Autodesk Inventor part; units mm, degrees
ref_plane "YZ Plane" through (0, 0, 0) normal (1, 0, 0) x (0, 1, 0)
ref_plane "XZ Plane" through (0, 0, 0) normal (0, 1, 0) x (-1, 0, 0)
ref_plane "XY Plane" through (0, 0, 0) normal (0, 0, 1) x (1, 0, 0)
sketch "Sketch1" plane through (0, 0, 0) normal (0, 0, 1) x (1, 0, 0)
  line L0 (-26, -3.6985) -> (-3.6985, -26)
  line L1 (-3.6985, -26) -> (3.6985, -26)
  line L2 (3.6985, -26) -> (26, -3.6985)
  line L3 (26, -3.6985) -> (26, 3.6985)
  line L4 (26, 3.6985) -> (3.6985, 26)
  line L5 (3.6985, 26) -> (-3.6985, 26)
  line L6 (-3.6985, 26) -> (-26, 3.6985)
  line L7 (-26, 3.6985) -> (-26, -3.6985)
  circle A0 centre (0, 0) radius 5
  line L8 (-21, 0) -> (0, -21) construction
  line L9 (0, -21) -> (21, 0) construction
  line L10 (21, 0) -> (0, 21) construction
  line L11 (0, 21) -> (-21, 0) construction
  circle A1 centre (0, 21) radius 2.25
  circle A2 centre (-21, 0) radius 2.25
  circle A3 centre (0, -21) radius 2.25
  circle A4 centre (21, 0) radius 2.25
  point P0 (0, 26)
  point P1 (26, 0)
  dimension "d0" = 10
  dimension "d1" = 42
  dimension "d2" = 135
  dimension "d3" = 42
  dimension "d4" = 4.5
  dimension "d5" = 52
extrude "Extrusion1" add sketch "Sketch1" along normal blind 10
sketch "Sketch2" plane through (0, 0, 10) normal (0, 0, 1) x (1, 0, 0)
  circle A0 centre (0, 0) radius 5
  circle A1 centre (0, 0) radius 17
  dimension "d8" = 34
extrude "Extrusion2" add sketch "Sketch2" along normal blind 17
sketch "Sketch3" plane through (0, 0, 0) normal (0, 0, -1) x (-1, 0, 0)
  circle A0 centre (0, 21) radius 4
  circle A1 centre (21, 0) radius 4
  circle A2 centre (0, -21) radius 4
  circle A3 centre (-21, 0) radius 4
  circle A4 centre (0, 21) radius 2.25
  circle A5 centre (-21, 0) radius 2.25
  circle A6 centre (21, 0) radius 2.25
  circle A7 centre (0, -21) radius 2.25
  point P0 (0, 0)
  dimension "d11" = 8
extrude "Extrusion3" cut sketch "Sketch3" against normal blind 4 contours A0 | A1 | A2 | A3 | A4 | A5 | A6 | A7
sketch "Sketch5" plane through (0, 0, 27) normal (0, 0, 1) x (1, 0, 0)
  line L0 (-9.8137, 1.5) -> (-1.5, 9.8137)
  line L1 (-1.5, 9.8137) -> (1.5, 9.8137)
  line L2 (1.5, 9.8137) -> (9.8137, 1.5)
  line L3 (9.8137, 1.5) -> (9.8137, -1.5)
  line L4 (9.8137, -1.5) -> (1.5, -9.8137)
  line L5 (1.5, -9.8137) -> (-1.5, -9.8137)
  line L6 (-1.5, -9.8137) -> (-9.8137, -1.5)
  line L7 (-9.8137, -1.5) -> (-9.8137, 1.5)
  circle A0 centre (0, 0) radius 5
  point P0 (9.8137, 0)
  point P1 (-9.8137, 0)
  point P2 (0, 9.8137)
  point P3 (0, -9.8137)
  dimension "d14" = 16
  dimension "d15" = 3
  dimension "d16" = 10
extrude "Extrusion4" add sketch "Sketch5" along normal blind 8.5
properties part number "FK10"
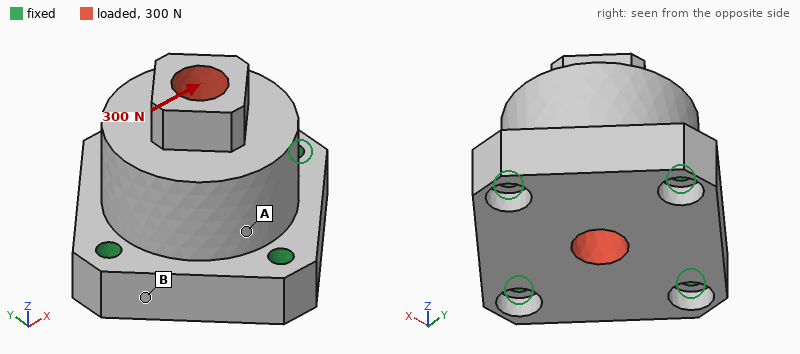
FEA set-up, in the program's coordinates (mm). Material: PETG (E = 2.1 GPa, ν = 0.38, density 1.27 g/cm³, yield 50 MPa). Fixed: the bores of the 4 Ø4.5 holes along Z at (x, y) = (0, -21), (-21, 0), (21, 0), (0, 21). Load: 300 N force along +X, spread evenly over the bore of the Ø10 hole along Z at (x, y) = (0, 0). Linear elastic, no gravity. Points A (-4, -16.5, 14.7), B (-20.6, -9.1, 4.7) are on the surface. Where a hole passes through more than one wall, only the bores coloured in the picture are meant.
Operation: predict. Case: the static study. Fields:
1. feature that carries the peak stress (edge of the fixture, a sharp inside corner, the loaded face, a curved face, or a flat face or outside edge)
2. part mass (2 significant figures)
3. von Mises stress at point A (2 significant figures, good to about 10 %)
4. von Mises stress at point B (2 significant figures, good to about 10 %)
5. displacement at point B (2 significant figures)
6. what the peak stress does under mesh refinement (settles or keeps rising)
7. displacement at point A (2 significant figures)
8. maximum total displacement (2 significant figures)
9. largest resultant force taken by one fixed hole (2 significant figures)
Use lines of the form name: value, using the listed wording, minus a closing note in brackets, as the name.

feature that carries the peak stress: edge of the fixture
part mass: 39 g
von Mises stress at point A: 0.35 MPa
von Mises stress at point B: 0.65 MPa
displacement at point B: 6.0 µm
what the peak stress does under mesh refinement: keeps rising
displacement at point A: 8.5 µm
maximum total displacement: 31 µm
largest resultant force taken by one fixed hole: 130 N
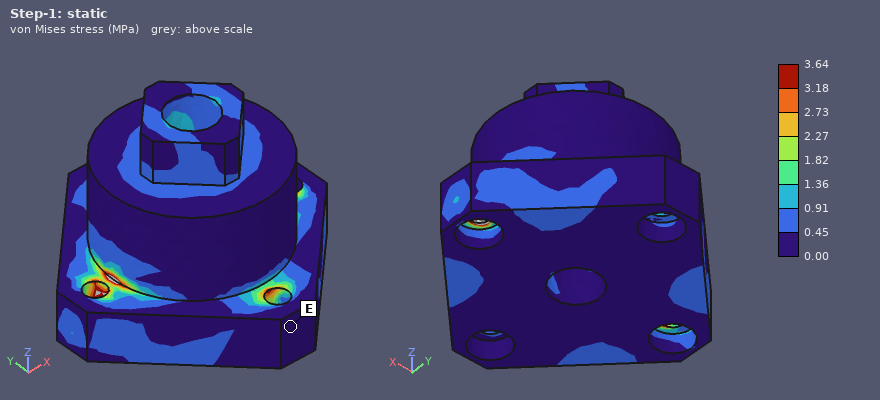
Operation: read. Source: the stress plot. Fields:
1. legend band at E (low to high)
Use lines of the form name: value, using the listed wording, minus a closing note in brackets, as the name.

legend band at E: 0.00 to 0.45 MPa
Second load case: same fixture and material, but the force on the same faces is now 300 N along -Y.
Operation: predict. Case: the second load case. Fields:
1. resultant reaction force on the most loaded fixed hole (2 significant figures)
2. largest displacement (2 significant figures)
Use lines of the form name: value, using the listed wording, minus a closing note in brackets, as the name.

resultant reaction force on the most loaded fixed hole: 130 N
largest displacement: 31 µm
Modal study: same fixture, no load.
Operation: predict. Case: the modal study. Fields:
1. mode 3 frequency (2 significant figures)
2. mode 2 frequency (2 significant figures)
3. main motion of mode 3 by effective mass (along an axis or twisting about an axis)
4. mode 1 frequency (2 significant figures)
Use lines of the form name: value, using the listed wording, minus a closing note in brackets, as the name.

mode 3 frequency: 5200 Hz
mode 2 frequency: 4300 Hz
main motion of mode 3 by effective mass: along Z
mode 1 frequency: 4300 Hz
